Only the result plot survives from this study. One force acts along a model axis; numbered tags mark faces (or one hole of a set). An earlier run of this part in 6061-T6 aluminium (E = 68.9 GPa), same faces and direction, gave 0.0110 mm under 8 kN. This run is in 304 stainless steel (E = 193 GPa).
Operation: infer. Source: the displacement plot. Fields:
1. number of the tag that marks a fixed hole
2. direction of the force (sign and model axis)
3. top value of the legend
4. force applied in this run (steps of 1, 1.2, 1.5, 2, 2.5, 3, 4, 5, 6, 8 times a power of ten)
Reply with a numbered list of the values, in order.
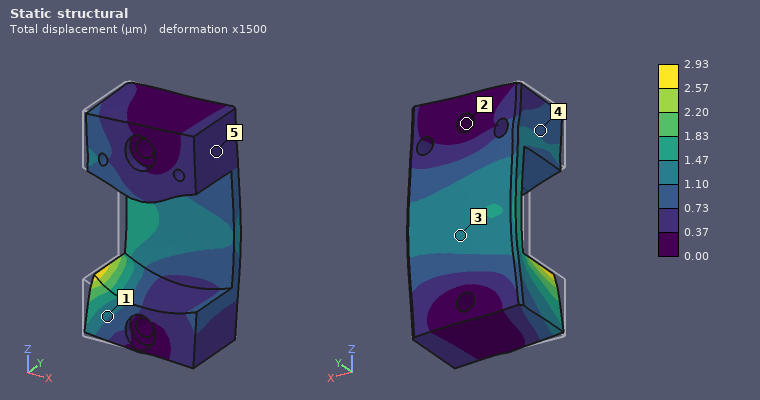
1. 2
2. +X
3. 2.93 µm
4. 6 kN
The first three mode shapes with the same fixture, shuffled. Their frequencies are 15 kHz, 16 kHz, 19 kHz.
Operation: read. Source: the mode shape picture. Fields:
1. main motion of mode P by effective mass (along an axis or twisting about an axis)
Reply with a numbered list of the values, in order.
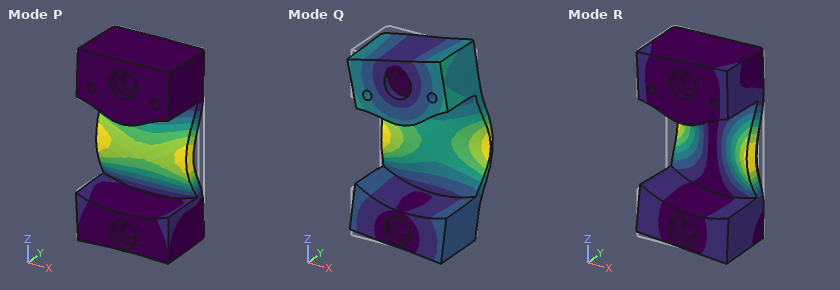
1. along Y
